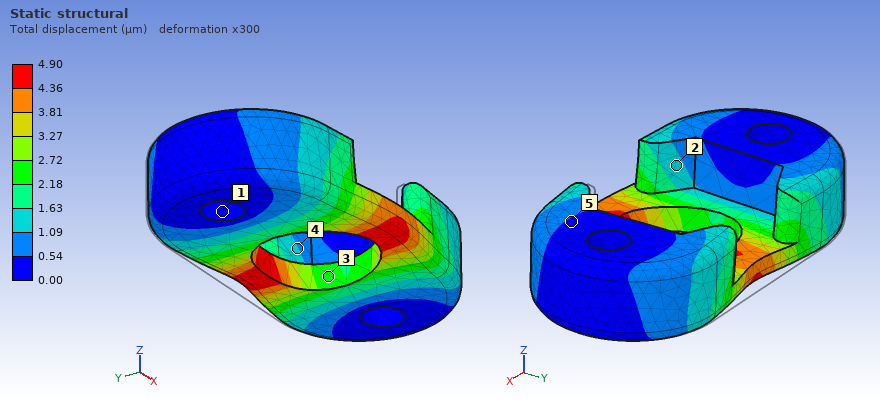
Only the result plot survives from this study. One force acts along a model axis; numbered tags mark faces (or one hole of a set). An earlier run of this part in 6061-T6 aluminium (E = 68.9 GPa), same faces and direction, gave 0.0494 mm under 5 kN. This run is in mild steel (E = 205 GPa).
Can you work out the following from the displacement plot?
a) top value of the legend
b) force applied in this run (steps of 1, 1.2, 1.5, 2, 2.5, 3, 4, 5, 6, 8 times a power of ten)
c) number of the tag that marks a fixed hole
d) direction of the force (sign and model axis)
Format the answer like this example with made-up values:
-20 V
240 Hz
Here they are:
4.90 µm
1.5 kN
1
-Y
